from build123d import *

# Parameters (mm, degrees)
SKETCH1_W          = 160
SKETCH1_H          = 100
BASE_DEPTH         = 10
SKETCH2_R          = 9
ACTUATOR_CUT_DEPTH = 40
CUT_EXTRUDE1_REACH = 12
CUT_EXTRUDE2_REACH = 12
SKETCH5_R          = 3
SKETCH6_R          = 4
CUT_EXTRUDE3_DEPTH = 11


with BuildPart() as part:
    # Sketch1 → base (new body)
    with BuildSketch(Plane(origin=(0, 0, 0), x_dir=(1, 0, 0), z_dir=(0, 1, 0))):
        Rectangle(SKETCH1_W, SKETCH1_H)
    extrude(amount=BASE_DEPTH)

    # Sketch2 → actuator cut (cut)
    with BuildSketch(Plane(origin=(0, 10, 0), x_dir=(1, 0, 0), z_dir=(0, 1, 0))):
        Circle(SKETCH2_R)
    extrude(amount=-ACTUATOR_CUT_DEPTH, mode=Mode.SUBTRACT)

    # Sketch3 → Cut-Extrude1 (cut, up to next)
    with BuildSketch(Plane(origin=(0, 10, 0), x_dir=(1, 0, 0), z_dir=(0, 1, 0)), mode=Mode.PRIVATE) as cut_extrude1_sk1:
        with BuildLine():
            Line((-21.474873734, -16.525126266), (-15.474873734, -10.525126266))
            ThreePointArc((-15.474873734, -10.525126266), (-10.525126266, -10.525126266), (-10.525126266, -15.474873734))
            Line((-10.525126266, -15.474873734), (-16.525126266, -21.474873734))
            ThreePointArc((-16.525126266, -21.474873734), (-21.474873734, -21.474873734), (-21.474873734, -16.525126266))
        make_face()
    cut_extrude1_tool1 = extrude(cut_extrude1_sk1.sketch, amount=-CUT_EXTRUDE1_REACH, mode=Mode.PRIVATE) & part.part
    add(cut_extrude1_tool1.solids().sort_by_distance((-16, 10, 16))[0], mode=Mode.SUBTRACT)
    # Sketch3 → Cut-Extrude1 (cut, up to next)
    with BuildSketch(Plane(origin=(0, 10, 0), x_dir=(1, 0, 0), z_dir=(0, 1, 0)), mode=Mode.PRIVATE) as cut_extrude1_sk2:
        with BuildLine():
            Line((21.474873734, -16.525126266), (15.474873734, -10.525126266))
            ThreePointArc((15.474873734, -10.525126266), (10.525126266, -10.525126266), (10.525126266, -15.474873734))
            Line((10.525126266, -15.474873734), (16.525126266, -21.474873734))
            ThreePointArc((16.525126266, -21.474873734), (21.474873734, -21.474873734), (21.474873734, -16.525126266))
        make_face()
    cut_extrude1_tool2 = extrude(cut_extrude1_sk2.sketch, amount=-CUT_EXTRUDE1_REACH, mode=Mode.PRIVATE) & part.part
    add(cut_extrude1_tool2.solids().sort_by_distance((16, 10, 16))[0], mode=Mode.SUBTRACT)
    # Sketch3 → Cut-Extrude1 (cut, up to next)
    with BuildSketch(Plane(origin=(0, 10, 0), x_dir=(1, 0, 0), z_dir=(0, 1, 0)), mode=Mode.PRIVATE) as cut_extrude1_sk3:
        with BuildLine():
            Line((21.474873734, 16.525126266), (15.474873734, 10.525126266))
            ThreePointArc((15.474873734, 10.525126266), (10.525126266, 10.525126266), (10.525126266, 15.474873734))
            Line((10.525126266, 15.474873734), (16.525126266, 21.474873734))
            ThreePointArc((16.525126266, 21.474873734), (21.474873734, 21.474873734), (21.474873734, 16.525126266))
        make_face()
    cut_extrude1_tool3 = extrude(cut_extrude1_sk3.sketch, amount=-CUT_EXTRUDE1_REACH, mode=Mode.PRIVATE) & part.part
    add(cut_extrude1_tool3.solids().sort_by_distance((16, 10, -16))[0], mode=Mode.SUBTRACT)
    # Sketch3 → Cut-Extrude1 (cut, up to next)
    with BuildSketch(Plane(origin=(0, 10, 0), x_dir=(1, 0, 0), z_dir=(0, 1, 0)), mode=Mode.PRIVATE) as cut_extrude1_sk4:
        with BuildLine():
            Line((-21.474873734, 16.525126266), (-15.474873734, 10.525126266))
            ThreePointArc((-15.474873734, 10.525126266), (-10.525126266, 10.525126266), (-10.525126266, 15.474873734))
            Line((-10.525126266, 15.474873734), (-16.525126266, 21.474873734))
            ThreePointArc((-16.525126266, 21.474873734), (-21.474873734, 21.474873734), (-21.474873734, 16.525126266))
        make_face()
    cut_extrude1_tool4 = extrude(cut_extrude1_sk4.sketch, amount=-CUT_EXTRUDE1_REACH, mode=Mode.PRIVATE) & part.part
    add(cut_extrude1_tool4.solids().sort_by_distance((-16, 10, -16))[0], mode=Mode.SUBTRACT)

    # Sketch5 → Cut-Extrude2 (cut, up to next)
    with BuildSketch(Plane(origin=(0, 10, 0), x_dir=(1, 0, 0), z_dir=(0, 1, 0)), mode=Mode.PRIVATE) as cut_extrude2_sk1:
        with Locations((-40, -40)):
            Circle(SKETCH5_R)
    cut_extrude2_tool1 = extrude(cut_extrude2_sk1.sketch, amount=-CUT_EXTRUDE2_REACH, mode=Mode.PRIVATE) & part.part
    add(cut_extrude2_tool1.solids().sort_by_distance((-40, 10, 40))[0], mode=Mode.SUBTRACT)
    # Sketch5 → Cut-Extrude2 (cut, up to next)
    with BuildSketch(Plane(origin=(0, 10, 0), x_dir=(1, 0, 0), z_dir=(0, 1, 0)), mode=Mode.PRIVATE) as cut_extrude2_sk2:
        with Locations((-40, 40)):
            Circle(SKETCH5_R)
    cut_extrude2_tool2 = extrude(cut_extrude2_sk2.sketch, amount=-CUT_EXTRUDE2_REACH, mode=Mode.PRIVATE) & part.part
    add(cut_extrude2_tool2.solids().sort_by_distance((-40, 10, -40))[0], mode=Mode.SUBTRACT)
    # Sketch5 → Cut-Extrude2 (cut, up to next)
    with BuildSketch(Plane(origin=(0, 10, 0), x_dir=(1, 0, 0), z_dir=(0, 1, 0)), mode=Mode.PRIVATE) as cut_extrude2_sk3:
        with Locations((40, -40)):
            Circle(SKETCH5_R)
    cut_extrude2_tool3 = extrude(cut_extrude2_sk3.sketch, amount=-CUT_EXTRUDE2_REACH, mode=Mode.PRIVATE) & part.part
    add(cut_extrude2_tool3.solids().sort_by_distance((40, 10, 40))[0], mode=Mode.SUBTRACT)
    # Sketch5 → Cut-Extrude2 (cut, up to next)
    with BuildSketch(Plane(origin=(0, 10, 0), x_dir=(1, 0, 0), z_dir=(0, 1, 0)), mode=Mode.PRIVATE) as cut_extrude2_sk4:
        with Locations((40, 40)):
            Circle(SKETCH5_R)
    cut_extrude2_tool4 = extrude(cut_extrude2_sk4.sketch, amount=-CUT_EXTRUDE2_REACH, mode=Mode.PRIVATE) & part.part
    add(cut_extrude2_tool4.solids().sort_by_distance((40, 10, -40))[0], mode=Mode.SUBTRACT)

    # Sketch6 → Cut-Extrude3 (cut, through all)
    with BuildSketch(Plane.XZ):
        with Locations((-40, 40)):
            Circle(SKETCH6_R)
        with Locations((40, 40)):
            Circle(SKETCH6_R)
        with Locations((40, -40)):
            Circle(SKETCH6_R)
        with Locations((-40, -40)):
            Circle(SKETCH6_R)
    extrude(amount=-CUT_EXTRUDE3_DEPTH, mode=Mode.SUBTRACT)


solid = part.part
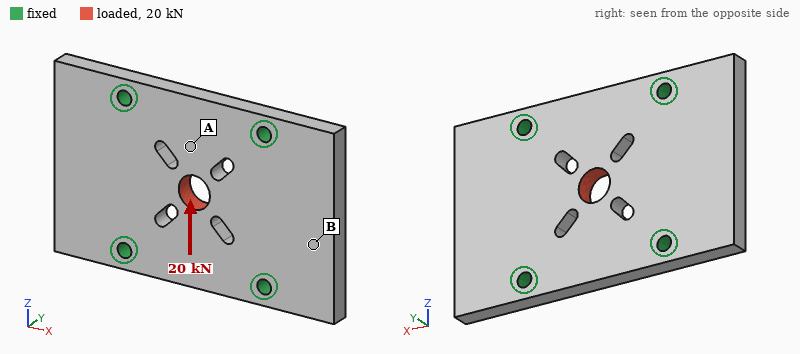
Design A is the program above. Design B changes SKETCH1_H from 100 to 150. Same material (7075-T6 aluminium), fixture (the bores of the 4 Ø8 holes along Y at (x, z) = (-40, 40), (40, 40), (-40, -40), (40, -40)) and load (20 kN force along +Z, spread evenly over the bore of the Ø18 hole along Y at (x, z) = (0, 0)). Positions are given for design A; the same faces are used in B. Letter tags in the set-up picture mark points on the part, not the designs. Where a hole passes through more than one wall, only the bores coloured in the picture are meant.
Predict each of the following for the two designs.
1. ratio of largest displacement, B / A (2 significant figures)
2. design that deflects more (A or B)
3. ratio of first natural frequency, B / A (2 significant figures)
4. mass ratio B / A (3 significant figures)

0.84
A
0.99
1.53
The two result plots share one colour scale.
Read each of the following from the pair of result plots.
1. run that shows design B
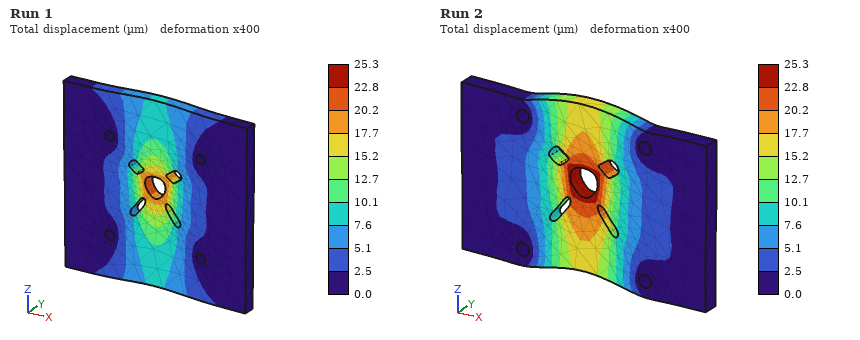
Run 1
